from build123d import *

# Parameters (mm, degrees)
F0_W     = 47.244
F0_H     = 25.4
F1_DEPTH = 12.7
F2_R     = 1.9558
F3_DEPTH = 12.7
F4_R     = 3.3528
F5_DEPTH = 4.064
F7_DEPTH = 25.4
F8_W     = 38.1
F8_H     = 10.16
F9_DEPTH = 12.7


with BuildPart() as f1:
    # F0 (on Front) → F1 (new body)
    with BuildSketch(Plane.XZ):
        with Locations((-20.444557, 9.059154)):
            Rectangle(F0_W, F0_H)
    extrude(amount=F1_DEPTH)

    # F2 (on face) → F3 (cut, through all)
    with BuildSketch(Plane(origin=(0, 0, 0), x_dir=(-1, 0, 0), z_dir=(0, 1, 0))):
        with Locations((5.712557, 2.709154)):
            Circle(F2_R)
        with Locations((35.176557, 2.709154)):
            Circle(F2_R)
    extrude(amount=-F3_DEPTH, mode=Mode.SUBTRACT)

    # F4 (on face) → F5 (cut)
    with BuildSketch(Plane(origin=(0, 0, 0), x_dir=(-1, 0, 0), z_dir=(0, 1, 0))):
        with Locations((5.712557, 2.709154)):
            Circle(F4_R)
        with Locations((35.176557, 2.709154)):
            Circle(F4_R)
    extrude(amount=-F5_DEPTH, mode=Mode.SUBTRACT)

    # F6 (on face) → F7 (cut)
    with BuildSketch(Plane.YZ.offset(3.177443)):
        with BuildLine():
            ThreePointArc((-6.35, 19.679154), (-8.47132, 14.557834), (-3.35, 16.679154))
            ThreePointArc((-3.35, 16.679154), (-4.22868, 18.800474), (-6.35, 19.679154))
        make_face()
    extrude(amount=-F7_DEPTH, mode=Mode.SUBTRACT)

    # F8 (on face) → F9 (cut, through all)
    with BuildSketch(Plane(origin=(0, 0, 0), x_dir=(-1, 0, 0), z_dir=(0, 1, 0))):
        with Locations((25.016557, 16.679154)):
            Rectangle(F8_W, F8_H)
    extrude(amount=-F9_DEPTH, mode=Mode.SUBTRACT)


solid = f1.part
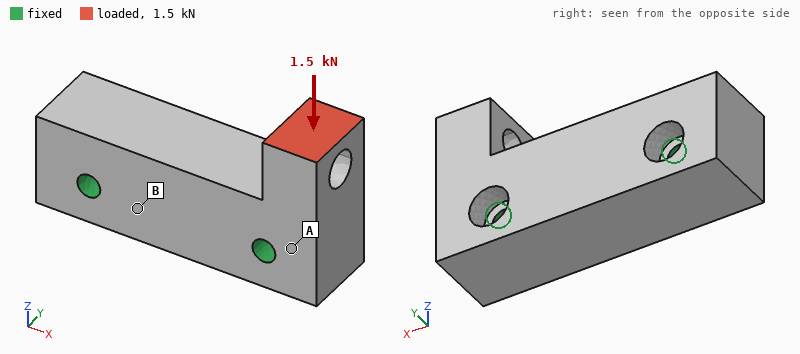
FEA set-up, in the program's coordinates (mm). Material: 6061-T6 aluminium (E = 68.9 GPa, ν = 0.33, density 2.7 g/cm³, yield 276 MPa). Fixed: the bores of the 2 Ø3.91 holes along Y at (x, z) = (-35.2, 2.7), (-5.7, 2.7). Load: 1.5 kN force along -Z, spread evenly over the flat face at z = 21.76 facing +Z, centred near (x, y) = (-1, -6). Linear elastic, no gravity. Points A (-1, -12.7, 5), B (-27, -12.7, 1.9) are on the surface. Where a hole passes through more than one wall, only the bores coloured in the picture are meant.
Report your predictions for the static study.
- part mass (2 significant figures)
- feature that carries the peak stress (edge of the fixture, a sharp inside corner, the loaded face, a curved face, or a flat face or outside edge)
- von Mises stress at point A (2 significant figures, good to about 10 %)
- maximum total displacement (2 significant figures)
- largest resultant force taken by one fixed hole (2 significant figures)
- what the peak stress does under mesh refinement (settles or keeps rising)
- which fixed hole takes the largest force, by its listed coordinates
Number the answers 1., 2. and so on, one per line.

1. 26 g
2. edge of the fixture
3. 12 MPa
4. 14 µm
5. 1.6 kN
6. keeps rising
7. (-5.7, 2.7)
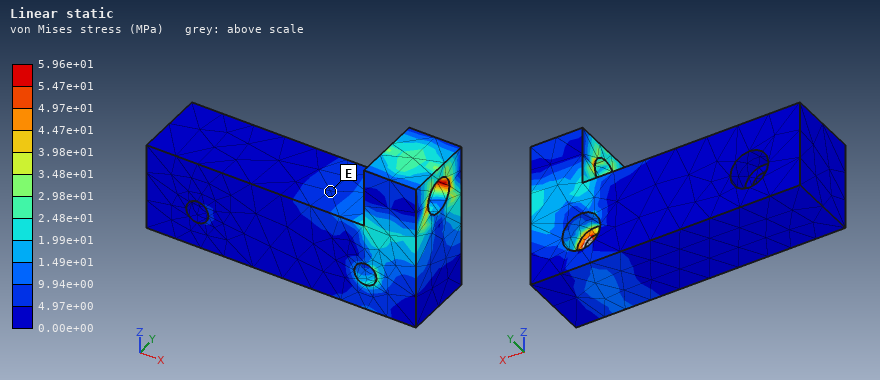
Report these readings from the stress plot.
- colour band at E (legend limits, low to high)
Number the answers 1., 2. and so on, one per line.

1. 4.97e+00 to 9.94e+00 MPa
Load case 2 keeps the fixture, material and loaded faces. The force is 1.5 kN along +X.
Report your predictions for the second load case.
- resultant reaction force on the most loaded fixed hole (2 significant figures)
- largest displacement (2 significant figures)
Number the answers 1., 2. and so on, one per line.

1. 1.1 kN
2. 70 µm
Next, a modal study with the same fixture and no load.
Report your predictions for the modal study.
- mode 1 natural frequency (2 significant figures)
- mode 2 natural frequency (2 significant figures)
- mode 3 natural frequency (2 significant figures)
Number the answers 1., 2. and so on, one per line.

1. 19 kHz
2. 22 kHz
3. 31 kHz
